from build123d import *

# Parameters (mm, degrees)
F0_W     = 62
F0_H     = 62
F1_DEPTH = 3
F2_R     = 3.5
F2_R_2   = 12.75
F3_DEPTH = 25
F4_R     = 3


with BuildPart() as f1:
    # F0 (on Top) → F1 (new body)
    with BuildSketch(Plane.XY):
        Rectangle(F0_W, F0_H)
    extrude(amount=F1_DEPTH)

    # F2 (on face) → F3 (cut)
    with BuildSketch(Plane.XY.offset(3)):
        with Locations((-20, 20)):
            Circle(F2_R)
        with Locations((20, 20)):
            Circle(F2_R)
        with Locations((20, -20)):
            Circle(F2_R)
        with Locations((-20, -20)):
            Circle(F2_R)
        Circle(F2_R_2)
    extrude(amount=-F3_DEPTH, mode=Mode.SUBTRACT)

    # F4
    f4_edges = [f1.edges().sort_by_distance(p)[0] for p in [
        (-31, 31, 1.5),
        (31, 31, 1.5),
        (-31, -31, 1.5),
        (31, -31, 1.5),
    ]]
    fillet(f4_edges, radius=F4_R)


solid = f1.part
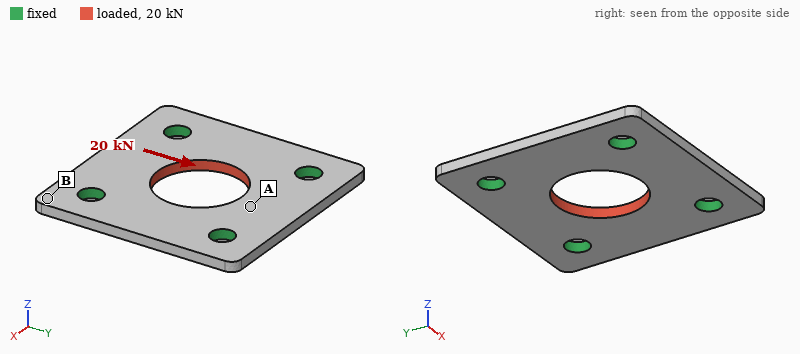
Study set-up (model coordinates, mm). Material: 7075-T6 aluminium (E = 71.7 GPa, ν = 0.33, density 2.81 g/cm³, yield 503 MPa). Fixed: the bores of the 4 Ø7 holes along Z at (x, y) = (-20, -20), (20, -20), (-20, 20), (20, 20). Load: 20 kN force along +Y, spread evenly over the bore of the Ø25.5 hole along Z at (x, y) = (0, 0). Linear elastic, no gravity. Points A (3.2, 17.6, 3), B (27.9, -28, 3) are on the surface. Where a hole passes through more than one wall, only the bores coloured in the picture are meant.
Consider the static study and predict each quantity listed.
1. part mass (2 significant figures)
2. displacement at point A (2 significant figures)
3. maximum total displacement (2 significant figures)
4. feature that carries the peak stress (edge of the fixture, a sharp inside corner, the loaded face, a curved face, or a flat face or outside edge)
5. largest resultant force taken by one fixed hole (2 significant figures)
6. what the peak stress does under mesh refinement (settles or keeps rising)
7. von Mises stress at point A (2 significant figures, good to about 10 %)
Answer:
27 g
34 µm
40 µm
edge of the fixture
5.2 kN
keeps rising
65 MPa
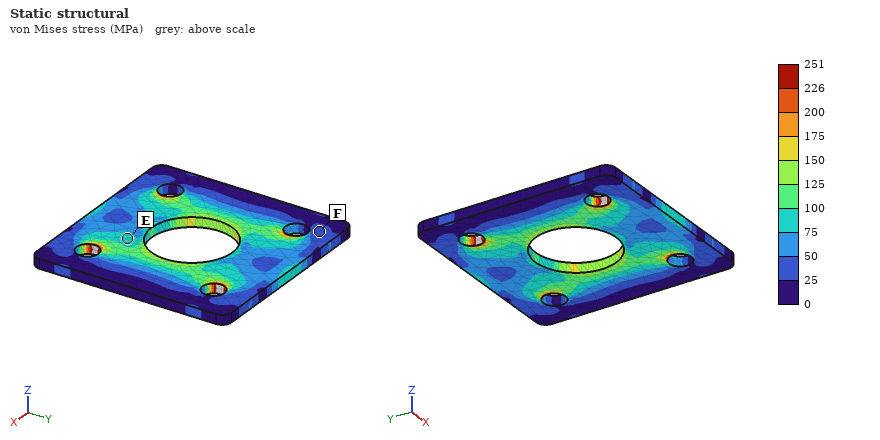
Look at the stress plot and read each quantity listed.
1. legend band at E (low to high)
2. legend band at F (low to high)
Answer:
75 to 100 MPa
25 to 50 MPa
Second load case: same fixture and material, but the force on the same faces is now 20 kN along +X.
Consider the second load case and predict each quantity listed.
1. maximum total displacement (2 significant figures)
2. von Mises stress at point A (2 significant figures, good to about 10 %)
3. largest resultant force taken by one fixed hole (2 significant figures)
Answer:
40 µm
89 MPa
5.2 kN
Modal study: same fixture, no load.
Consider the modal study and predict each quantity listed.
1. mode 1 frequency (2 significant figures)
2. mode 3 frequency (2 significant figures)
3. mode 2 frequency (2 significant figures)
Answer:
11 kHz
11 kHz
11 kHz
